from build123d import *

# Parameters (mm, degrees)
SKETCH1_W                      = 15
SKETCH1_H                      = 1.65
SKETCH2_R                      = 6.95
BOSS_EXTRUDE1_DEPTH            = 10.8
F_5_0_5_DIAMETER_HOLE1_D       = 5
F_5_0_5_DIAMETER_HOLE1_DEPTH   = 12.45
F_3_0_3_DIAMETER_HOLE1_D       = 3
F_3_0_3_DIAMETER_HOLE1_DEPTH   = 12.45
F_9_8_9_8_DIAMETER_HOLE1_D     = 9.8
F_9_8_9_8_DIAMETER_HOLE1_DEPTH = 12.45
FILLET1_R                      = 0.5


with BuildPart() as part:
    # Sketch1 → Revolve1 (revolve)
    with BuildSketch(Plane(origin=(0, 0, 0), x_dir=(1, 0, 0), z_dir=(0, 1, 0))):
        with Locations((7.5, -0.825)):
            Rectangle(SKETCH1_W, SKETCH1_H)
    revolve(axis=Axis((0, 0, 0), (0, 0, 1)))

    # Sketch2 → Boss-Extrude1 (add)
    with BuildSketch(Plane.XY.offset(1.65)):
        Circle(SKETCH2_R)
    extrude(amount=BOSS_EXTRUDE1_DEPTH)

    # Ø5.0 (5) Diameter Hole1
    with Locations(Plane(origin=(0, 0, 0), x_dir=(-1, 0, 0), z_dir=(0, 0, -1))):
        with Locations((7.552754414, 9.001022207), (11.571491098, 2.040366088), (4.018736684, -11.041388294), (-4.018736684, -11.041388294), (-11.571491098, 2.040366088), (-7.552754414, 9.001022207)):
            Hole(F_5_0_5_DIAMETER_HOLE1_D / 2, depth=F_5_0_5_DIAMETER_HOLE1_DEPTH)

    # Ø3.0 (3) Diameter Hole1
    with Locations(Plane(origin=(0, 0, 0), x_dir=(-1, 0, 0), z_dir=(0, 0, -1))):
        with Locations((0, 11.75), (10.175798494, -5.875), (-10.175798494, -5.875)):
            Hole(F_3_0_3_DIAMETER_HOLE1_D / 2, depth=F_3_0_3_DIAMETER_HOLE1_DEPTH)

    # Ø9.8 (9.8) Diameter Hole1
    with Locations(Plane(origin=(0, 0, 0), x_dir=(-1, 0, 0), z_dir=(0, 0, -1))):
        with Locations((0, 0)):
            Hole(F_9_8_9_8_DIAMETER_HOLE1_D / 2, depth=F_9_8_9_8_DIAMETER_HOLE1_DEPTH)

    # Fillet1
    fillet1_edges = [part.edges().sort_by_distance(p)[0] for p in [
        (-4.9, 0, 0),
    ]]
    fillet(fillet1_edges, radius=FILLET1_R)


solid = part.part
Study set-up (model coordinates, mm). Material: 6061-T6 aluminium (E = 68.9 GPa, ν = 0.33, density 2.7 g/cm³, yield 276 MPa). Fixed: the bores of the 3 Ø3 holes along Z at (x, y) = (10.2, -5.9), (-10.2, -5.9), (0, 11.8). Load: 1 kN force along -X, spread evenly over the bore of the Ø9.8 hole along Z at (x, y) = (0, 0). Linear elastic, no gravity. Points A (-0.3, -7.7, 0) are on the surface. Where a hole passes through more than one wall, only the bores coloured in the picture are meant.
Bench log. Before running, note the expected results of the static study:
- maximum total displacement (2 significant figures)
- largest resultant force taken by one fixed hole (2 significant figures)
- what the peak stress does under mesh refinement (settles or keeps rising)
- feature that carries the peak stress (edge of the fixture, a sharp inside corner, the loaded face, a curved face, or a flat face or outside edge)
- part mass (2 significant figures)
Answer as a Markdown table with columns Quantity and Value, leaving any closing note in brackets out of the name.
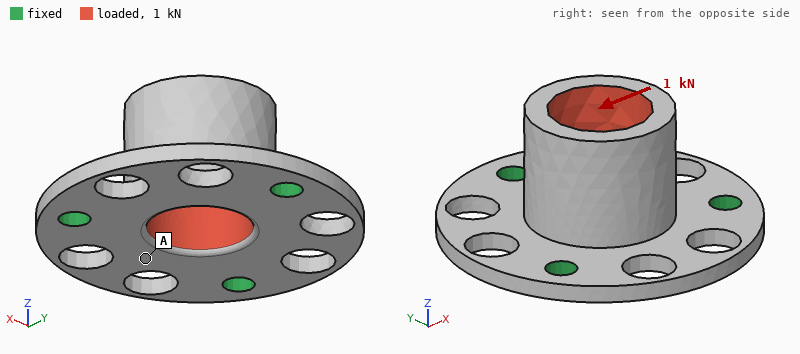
| Quantity | Value |
|---|---|
| maximum total displacement | 48 µm |
| largest resultant force taken by one fixed hole | 500 N |
| what the peak stress does under mesh refinement | keeps rising |
| feature that carries the peak stress | edge of the fixture |
| part mass | 4.4 g |
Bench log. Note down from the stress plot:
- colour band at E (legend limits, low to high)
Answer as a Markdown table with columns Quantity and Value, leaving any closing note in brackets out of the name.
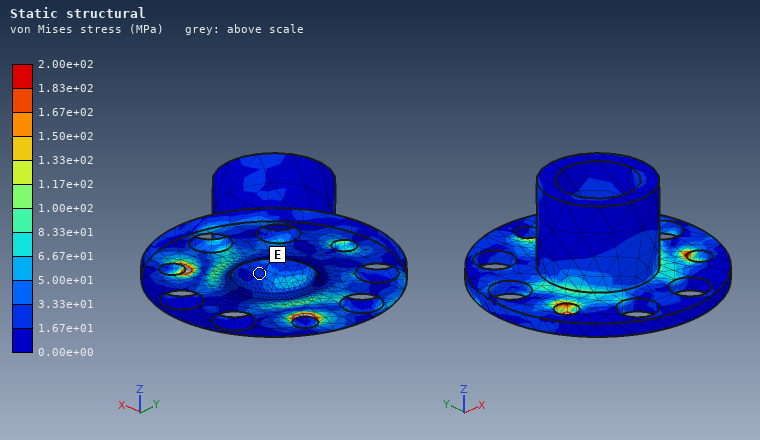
| Quantity | Value |
|---|---|
| colour band at E | 1.67e+01 to 3.33e+01 MPa |
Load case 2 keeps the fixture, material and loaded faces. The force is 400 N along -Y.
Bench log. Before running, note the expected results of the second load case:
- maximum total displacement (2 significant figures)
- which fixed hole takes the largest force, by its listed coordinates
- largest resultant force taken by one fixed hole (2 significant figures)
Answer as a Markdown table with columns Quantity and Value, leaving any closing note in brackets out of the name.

| Quantity | Value |
|---|---|
| maximum total displacement | 20 µm |
| which fixed hole takes the largest force, by its listed coordinates | (0, 11.8) |
| largest resultant force taken by one fixed hole | 220 N |
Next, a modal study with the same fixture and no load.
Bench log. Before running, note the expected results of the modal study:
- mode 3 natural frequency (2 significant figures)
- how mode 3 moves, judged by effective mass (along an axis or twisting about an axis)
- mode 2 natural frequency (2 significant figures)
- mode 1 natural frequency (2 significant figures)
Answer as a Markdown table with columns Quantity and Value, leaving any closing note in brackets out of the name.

| Quantity | Value |
|---|---|
| mode 3 natural frequency | 18 kHz |
| how mode 3 moves, judged by effective mass | along Z |
| mode 2 natural frequency | 15 kHz |
| mode 1 natural frequency | 15 kHz |
